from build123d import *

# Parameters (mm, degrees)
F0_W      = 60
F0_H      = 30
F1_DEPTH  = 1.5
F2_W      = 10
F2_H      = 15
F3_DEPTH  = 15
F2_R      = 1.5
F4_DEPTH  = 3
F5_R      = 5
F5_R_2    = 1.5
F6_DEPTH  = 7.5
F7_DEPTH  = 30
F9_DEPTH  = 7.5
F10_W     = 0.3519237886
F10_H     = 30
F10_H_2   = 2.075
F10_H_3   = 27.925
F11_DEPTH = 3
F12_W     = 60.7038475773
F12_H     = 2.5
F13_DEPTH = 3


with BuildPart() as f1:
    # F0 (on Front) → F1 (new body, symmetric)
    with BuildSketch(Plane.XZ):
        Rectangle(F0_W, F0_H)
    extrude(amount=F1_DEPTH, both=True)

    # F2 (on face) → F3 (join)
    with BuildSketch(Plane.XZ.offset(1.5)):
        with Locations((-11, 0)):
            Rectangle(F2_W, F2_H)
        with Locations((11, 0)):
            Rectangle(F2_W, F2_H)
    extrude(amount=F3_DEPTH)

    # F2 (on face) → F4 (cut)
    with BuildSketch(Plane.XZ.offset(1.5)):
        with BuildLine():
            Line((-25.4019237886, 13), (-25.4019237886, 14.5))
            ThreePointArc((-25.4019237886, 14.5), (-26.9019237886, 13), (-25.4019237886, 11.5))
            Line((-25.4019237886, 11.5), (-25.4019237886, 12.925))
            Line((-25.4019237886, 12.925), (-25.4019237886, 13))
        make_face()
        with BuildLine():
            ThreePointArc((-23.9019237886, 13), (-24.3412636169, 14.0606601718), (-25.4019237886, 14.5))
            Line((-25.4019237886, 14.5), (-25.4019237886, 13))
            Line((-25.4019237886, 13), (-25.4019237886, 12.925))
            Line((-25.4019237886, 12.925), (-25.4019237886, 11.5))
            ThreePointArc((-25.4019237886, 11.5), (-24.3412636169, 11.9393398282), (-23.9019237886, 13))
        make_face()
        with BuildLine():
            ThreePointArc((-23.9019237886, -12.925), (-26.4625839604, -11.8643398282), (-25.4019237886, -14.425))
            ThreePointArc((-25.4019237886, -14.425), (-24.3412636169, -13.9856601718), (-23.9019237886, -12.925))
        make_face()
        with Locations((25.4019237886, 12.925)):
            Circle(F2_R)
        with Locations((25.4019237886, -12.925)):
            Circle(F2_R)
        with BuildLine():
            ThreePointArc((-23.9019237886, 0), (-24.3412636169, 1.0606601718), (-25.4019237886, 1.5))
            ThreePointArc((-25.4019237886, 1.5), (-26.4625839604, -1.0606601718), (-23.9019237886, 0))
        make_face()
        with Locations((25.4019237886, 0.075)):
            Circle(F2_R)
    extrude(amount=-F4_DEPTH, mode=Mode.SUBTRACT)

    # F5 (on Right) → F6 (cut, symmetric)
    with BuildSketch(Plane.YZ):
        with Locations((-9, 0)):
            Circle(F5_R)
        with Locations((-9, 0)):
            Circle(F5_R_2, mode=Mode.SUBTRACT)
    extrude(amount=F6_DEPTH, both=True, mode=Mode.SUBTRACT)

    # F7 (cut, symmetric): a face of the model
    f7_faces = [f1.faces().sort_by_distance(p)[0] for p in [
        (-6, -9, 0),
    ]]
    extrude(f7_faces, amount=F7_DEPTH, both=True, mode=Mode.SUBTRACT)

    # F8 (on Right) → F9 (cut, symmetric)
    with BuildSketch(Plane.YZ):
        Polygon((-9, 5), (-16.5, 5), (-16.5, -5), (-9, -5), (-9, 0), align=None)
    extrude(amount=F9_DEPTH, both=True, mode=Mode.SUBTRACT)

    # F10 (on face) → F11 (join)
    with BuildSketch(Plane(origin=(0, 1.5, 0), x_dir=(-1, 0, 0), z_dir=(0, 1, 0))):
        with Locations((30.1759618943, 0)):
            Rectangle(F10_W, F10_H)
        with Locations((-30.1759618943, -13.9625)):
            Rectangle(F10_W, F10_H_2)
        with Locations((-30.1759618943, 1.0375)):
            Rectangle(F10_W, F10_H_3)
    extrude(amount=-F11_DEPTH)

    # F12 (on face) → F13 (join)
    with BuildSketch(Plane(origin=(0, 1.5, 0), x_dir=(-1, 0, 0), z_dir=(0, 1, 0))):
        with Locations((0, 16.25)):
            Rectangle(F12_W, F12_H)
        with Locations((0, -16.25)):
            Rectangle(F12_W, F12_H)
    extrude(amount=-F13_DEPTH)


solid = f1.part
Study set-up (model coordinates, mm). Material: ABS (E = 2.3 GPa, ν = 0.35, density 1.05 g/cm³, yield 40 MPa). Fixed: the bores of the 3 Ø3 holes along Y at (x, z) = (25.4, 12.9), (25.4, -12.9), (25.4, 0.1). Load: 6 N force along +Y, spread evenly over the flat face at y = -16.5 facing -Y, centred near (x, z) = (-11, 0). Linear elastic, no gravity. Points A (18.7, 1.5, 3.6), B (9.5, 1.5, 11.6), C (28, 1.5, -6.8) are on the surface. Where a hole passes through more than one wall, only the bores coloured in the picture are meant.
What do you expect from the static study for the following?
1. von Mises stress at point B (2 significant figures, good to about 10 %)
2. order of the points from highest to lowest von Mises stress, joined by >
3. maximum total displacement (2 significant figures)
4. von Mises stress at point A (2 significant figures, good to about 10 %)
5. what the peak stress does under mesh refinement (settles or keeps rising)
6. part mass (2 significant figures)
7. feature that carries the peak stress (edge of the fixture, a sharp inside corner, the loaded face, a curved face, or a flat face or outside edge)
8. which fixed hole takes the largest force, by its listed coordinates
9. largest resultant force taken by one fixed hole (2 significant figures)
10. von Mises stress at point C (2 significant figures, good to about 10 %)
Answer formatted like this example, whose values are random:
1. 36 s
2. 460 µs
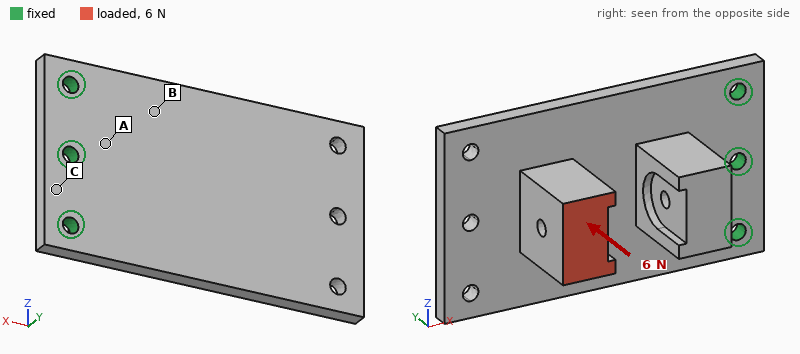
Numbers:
1. 1.4 MPa
2. A > B > C
3. 0.78 mm
4. 3.2 MPa
5. keeps rising
6. 11 g
7. edge of the fixture
8. (25.4, 0.1)
9. 3.4 N
10. 0.52 MPa
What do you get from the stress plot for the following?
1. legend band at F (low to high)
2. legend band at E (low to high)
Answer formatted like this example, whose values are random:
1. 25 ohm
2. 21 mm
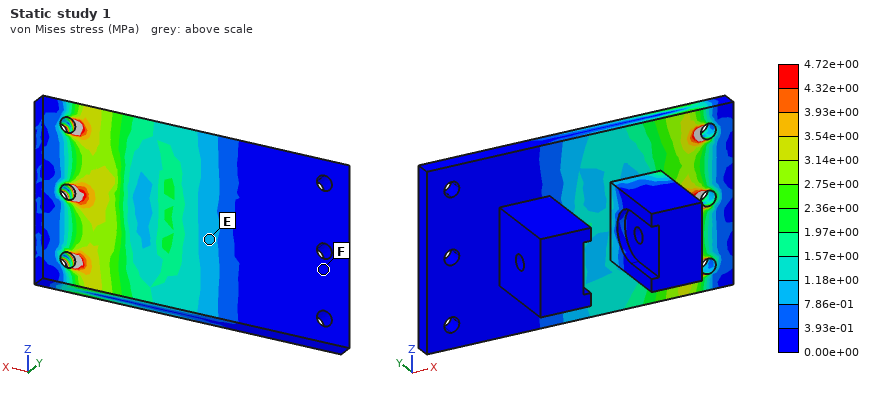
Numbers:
1. 0.00e+00 to 3.93e-01 MPa
2. 7.86e-01 to 1.18e+00 MPa
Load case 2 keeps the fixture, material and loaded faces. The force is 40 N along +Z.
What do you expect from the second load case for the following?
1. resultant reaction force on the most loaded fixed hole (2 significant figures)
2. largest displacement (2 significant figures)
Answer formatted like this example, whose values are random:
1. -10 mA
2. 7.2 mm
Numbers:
1. 62 N
2. 0.67 mm
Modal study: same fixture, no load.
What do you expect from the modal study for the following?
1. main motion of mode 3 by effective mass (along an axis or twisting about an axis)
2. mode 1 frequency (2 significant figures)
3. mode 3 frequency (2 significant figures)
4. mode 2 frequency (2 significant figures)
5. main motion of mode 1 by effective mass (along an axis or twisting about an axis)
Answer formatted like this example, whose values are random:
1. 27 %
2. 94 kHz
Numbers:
1. along Y
2. 210 Hz
3. 1100 Hz
4. 860 Hz
5. along Y
